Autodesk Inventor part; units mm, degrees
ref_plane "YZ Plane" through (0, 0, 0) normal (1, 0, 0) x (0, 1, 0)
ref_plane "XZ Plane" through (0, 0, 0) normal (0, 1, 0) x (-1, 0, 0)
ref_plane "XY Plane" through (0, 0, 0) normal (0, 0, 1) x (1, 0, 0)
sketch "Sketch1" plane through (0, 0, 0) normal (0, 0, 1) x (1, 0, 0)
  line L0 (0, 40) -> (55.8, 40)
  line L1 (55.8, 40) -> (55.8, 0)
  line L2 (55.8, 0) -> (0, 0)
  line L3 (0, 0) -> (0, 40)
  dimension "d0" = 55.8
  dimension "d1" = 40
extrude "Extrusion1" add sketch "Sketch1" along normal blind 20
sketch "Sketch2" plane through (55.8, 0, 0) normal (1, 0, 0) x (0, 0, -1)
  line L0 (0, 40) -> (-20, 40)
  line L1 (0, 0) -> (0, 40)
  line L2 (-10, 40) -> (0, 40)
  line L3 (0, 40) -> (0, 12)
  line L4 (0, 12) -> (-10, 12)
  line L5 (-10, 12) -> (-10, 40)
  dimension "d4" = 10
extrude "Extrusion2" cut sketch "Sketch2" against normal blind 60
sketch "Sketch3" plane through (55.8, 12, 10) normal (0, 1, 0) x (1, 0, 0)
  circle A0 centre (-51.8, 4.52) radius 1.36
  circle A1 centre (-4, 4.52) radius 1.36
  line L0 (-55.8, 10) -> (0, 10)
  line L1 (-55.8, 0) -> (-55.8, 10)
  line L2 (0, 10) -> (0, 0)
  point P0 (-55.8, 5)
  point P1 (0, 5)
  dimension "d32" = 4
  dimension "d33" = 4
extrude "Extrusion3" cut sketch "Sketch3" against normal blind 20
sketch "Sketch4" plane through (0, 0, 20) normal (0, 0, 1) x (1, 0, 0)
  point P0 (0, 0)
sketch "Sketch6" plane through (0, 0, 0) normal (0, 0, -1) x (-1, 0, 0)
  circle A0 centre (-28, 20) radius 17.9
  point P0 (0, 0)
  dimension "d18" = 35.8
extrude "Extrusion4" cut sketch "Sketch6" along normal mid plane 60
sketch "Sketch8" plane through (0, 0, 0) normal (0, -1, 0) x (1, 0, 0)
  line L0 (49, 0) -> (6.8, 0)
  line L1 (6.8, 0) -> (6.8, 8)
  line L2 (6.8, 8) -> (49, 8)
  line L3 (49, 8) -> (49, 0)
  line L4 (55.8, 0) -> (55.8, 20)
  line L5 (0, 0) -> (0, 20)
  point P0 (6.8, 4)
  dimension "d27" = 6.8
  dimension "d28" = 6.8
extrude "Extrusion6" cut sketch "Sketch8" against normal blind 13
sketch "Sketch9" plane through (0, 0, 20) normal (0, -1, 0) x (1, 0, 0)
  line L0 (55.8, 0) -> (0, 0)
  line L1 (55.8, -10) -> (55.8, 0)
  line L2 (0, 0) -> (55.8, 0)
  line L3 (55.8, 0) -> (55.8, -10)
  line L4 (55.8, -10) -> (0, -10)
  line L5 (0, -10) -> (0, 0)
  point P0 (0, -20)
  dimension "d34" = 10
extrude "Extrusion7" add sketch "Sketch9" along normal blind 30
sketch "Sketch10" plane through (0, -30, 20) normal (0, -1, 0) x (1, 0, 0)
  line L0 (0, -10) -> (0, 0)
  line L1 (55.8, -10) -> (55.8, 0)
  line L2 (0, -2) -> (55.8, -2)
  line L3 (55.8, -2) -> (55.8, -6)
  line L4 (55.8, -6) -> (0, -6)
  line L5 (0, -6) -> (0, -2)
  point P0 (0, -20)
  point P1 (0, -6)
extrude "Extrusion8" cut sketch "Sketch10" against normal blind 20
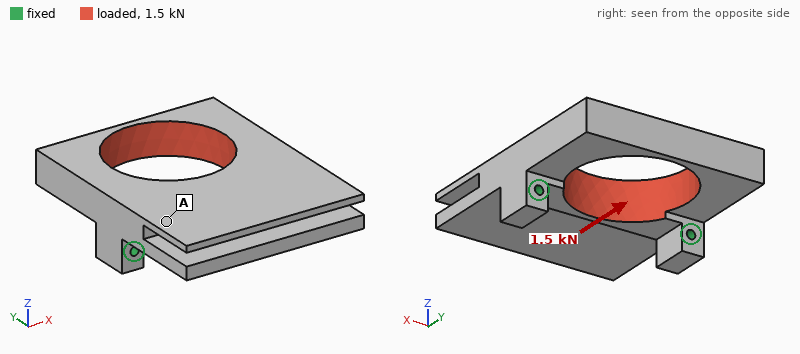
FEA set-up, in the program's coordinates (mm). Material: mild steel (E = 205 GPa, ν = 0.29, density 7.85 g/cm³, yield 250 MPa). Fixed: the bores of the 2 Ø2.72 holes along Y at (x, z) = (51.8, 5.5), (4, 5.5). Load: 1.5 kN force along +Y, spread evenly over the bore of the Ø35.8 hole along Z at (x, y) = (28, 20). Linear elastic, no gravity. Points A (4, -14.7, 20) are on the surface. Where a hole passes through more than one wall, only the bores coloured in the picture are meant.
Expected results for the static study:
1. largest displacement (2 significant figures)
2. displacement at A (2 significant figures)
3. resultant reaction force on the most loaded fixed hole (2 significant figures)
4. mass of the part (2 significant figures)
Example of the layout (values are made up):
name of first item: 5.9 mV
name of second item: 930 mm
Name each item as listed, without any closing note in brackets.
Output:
largest displacement: 8.5 µm
displacement at A: 4.2 µm
resultant reaction force on the most loaded fixed hole: 750 N
mass of the part: 210 g
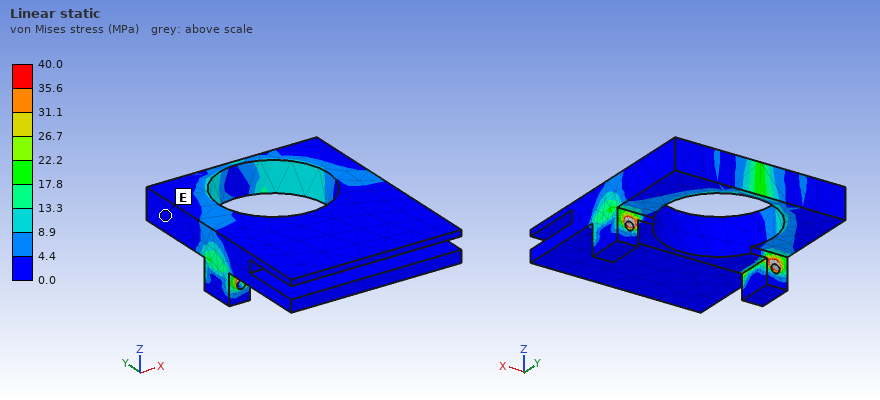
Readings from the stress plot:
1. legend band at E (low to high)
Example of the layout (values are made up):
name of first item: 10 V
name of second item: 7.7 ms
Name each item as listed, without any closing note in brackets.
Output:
legend band at E: 0.0 to 4.4 MPa
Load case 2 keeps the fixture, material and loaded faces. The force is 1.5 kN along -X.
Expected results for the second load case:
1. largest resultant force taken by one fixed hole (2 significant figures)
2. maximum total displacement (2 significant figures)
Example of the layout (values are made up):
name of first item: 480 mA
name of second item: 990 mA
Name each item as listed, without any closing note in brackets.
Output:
largest resultant force taken by one fixed hole: 850 N
maximum total displacement: 12 µm
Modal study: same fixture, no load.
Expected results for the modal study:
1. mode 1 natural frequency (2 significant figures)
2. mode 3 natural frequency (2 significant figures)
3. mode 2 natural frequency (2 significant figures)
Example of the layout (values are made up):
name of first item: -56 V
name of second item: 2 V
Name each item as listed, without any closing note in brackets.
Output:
mode 1 natural frequency: 3100 Hz
mode 3 natural frequency: 4900 Hz
mode 2 natural frequency: 4300 Hz
